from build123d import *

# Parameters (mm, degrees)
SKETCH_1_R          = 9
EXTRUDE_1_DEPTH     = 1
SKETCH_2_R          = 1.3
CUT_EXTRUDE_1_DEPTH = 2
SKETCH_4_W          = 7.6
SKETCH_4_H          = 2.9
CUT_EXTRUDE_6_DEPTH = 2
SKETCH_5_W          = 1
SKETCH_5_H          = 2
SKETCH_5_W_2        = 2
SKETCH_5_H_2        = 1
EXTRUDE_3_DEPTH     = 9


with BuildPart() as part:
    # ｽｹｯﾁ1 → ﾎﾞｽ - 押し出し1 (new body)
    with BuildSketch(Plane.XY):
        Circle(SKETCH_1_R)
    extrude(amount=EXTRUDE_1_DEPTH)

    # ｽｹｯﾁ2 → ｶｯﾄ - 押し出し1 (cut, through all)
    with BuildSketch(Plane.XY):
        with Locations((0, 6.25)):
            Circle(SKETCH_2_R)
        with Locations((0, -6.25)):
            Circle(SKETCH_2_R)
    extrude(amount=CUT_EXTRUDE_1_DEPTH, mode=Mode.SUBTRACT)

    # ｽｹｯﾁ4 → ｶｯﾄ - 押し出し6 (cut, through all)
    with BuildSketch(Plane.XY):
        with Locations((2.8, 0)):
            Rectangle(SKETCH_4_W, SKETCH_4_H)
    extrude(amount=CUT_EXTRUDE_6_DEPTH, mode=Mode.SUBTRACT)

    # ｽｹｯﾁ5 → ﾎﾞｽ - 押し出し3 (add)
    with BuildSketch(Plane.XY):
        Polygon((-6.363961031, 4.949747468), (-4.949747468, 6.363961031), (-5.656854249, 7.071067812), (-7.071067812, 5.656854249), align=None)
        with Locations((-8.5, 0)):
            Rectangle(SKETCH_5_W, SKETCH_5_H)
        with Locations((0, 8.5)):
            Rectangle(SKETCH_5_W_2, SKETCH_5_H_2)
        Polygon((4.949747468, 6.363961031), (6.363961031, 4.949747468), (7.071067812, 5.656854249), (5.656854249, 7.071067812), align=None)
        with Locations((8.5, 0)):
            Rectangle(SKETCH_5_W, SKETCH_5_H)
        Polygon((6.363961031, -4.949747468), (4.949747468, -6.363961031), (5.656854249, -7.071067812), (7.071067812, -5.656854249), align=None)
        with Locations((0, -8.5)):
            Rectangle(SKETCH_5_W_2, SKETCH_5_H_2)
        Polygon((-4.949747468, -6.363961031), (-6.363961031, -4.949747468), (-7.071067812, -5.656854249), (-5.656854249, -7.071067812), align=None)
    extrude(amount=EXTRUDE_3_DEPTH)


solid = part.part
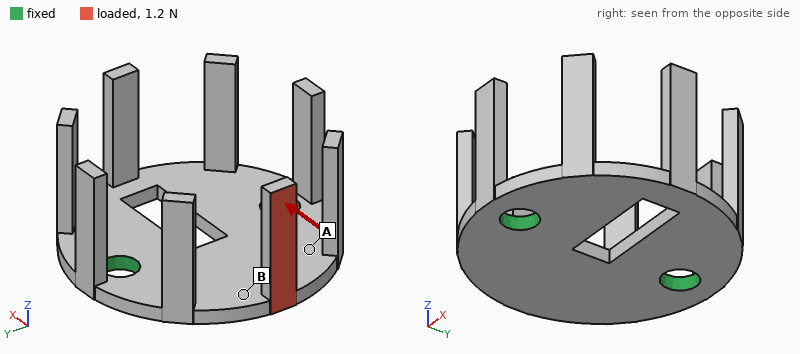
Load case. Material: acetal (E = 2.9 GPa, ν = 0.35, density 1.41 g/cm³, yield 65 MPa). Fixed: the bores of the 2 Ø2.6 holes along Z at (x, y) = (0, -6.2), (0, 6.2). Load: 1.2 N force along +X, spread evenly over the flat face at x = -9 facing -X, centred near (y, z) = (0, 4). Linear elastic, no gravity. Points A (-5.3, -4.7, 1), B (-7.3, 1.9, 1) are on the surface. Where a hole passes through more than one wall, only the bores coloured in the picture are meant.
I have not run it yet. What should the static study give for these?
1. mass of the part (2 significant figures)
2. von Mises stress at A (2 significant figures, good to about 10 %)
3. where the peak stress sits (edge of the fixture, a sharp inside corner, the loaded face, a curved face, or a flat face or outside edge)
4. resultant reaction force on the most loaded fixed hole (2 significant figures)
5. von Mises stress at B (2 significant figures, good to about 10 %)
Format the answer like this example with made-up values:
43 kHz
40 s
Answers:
0.49 g
1.7 MPa
the loaded face
0.67 N
3.6 MPa
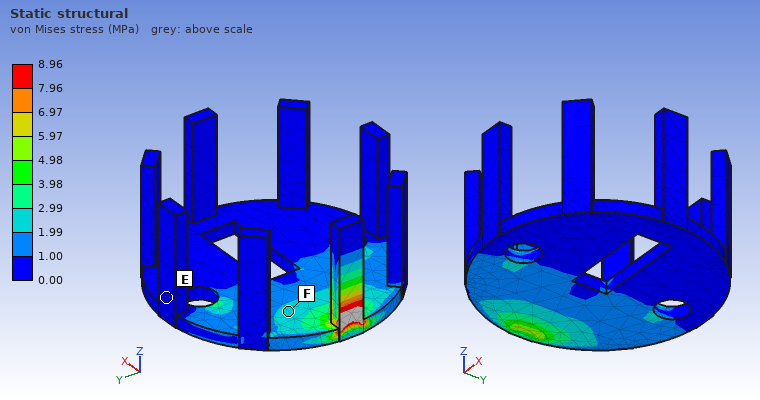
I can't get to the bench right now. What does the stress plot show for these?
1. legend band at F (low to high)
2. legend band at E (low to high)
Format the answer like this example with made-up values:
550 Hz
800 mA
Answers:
1.99 to 2.99 MPa
0.00 to 1.00 MPa
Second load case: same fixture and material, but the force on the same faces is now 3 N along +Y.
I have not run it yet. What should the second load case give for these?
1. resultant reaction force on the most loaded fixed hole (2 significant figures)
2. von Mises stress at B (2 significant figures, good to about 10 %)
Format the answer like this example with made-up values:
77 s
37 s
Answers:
2.7 N
7.6 MPa
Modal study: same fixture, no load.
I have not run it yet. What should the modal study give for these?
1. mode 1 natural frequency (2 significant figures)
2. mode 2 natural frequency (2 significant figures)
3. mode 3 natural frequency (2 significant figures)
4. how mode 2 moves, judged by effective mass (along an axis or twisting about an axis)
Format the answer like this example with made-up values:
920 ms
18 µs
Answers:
1900 Hz
1900 Hz
2500 Hz
along Z
